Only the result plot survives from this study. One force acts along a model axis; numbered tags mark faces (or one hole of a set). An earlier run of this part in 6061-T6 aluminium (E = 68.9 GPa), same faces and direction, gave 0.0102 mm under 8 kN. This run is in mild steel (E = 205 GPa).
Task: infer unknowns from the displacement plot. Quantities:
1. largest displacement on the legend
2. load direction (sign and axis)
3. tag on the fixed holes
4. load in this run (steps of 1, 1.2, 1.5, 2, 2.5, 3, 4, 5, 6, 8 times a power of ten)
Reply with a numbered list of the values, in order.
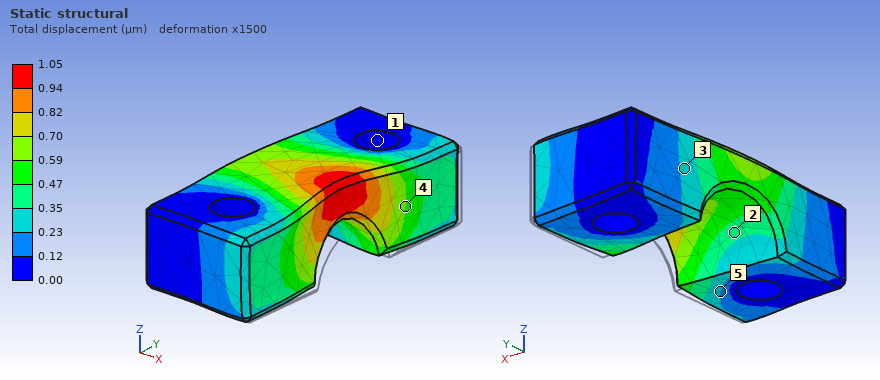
1. 1.05 µm
2. -X
3. 1
4. 2.5 kN
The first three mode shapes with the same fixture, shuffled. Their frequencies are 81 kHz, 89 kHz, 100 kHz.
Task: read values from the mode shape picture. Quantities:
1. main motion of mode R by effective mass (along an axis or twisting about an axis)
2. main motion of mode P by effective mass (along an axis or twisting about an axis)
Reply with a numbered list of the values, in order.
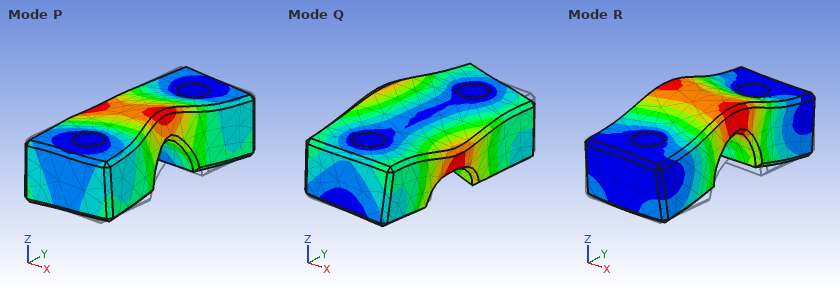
1. along Z
2. along X
